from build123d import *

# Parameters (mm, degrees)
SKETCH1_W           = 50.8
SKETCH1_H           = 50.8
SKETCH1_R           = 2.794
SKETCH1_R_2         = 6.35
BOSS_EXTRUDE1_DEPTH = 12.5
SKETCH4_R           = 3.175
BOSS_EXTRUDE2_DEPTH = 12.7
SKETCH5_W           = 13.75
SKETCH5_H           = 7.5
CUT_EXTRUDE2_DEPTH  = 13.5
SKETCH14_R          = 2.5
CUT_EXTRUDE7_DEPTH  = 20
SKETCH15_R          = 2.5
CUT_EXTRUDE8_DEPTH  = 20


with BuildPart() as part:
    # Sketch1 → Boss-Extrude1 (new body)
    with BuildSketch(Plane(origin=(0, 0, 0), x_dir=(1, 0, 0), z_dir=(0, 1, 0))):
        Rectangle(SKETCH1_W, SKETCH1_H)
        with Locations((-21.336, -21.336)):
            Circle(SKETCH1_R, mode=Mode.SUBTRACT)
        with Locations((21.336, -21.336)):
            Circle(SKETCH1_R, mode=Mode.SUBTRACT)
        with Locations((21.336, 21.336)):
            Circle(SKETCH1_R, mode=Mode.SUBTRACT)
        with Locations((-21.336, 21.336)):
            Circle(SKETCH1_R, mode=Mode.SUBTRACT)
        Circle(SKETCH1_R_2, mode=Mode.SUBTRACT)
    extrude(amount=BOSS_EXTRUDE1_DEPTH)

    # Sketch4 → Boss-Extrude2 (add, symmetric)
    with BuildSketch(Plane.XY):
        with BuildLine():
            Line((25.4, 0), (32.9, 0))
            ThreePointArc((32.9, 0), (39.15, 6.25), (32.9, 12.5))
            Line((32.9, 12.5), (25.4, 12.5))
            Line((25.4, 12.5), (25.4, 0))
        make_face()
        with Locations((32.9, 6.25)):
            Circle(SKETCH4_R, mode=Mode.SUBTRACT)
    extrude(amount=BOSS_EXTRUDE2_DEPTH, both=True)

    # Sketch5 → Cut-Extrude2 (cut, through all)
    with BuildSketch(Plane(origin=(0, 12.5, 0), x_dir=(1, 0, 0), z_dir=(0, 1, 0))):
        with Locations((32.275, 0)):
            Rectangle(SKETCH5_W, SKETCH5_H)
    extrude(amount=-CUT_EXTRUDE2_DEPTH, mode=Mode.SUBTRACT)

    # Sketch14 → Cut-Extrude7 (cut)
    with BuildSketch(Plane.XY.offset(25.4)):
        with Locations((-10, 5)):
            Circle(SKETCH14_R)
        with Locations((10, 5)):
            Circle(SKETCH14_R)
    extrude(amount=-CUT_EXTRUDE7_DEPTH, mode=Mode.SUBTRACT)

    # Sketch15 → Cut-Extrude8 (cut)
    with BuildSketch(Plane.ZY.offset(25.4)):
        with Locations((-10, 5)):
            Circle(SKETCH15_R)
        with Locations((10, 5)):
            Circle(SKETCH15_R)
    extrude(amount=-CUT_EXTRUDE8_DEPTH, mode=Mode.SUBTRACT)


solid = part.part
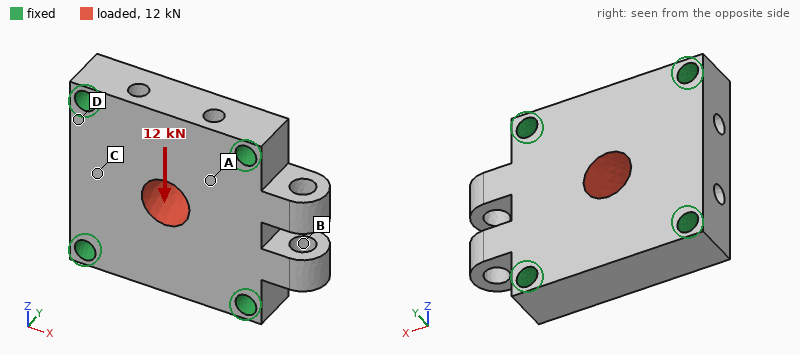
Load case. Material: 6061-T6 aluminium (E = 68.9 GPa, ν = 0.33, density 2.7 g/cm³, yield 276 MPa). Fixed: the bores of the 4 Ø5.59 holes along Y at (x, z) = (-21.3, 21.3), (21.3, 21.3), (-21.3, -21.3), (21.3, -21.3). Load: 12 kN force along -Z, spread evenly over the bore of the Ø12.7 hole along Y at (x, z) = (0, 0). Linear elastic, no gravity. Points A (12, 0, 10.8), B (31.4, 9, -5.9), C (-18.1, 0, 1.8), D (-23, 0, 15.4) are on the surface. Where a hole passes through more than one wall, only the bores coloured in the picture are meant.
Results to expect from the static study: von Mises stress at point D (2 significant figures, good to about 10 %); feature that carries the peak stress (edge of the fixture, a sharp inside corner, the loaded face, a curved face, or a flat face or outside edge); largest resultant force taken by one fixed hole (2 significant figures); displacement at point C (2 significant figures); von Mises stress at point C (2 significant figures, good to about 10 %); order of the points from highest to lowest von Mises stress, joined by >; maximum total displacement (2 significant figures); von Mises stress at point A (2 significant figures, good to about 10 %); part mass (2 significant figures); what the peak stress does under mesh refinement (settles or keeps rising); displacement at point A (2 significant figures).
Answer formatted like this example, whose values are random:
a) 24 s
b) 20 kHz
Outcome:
a) 15 MPa
b) edge of the fixture
c) 3.6 kN
d) 3.8 µm
e) 8.6 MPa
f) A > D > C > B
g) 11 µm
h) 27 MPa
i) 81 g
j) keeps rising
k) 4.9 µm
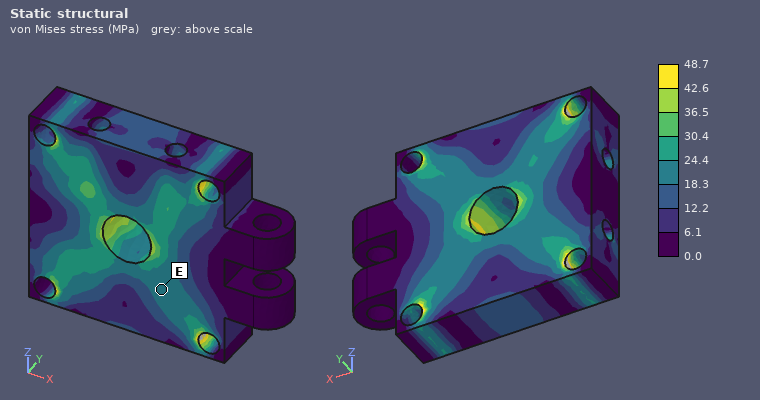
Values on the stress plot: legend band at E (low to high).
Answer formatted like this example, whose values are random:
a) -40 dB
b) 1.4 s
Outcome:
a) 18.3 to 24.4 MPa
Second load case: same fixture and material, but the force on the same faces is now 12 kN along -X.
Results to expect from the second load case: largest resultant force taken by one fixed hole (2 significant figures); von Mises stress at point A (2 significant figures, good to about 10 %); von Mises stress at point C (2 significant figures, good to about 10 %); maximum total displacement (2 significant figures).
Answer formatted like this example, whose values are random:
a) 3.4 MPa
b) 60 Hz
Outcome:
a) 3.6 kN
b) 27 MPa
c) 5.9 MPa
d) 11 µm
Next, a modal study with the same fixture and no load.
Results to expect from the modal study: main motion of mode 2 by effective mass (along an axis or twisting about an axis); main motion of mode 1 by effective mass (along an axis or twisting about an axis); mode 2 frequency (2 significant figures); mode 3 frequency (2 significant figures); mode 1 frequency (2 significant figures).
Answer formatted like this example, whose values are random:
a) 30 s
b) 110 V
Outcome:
a) along Y
b) along Y
c) 18 kHz
d) 22 kHz
e) 17 kHz
